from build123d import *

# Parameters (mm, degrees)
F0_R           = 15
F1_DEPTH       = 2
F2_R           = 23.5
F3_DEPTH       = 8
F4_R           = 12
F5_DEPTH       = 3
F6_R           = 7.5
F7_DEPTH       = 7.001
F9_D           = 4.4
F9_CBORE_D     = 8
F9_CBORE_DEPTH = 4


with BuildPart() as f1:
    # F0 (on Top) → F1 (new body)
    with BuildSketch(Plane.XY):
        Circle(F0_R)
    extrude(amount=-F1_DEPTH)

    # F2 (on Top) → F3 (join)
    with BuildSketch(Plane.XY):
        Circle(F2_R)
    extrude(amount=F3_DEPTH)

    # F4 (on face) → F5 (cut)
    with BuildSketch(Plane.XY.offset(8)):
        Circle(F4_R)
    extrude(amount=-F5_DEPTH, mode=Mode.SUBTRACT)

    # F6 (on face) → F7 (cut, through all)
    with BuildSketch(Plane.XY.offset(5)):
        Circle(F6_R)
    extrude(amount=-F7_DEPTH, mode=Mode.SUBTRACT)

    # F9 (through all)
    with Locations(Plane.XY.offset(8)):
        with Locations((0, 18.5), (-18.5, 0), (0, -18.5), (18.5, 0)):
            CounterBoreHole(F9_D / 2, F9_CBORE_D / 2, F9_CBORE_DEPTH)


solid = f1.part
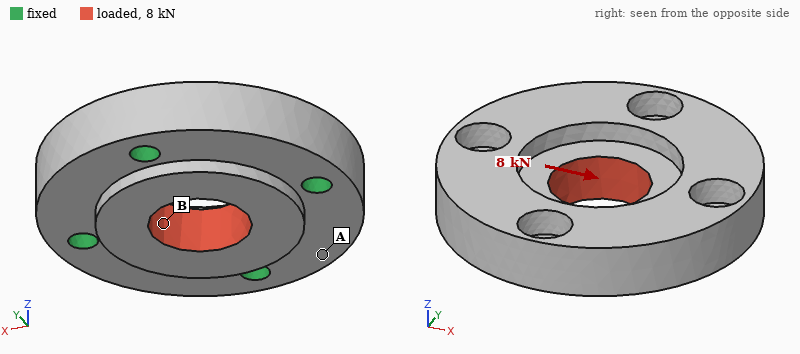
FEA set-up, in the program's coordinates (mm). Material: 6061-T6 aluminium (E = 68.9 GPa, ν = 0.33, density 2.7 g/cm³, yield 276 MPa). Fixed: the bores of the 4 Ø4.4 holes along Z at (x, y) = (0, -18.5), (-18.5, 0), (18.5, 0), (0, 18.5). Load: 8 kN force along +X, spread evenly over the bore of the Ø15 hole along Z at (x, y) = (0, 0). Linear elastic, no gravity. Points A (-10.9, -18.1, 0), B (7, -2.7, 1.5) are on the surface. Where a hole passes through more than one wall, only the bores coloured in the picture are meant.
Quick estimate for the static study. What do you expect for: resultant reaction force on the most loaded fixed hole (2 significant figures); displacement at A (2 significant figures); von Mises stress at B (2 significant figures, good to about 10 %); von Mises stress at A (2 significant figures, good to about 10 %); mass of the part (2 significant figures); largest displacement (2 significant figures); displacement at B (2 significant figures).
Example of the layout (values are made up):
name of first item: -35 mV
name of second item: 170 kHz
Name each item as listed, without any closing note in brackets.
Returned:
resultant reaction force on the most loaded fixed hole: 2.4 kN
displacement at A: 2.8 µm
von Mises stress at B: 29 MPa
von Mises stress at A: 12 MPa
mass of the part: 31 g
largest displacement: 7.6 µm
displacement at B: 6.4 µm
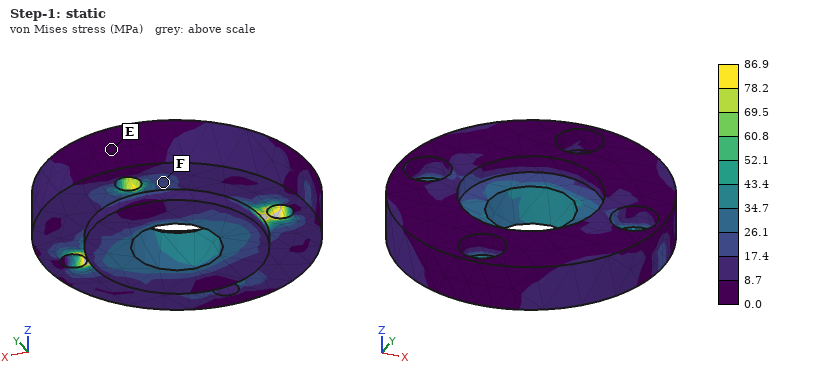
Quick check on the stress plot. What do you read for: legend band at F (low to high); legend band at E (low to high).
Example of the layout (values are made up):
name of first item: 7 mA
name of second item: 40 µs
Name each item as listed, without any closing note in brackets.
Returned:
legend band at F: 17.4 to 26.1 MPa
legend band at E: 0.0 to 8.7 MPa
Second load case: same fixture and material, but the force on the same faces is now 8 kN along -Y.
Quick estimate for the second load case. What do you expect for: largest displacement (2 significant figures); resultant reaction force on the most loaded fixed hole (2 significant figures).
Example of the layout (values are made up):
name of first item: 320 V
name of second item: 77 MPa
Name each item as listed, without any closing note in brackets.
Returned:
largest displacement: 7.6 µm
resultant reaction force on the most loaded fixed hole: 2.4 kN
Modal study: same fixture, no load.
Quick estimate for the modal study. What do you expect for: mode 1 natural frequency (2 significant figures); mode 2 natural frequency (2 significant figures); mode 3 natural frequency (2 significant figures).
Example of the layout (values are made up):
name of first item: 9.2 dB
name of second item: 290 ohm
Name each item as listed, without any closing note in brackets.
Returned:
mode 1 natural frequency: 22 kHz
mode 2 natural frequency: 26 kHz
mode 3 natural frequency: 26 kHz
